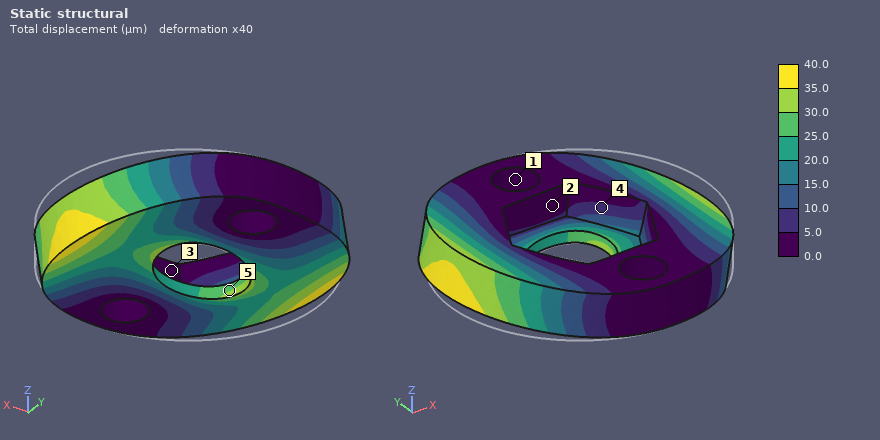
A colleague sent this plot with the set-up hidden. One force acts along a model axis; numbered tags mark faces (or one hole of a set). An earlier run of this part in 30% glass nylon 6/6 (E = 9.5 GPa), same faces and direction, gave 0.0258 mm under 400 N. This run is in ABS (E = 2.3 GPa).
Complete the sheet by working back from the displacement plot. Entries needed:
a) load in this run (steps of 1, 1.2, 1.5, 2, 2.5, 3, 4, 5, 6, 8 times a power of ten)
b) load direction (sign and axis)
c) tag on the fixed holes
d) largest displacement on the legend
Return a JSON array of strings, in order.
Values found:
["150 N", "-X", "1", "40.0 µm"]
